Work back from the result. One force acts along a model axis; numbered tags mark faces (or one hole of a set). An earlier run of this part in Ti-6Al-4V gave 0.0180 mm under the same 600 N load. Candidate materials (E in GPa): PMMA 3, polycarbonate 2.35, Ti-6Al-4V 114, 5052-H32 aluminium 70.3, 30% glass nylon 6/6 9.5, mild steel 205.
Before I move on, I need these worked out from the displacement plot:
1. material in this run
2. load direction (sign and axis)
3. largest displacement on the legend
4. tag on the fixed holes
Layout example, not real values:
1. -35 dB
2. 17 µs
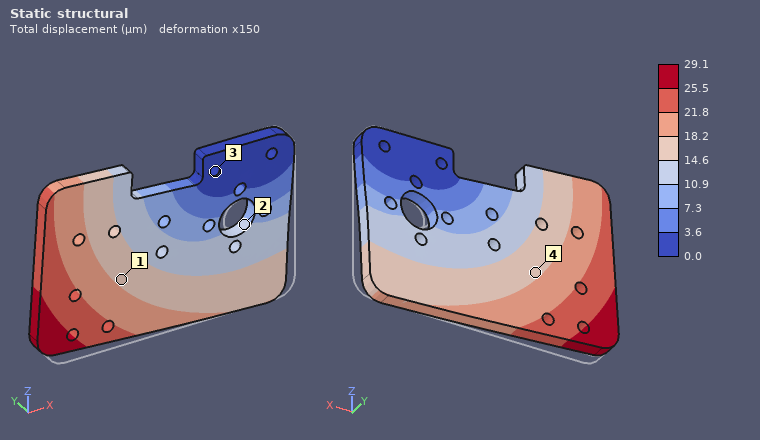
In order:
1. 5052-H32 aluminium
2. -X
3. 29.1 µm
4. 3
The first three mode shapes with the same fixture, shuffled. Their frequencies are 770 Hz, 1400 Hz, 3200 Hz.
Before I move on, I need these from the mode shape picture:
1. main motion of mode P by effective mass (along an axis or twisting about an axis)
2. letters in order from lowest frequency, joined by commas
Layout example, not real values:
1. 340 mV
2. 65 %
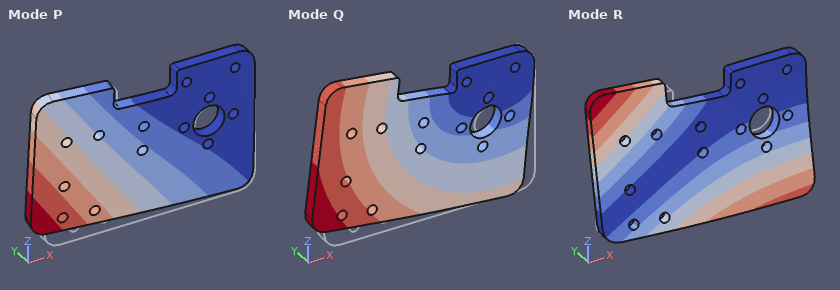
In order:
1. along Y
2. P, R, Q
